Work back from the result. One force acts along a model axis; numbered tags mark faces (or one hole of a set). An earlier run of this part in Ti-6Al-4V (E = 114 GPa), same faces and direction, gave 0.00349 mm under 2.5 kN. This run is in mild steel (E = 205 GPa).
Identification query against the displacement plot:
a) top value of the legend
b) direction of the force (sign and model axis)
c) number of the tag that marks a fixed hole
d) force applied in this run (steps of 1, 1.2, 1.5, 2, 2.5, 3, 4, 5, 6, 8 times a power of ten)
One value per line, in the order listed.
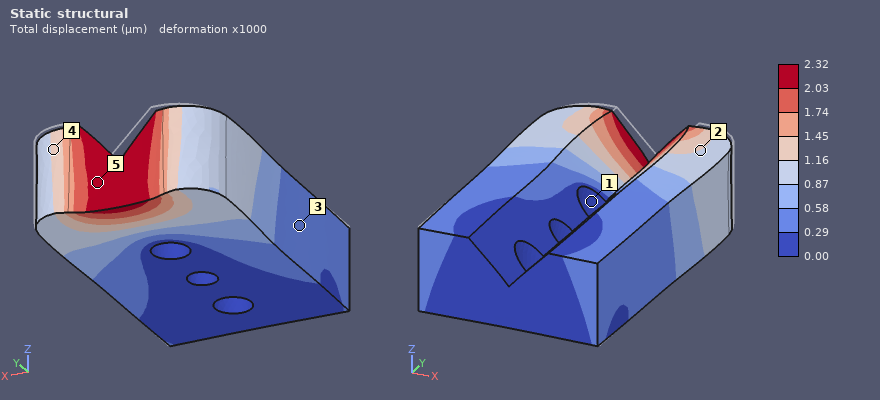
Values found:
2.32 µm
-Y
1
3 kN
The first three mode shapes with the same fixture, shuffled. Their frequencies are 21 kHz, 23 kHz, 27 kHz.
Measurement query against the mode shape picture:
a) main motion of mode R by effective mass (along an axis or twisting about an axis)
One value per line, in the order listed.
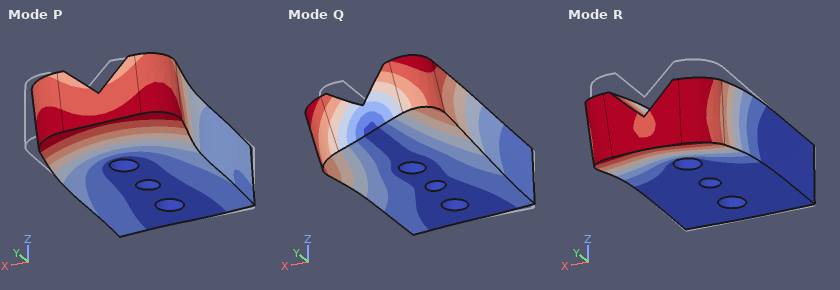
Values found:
along Z
